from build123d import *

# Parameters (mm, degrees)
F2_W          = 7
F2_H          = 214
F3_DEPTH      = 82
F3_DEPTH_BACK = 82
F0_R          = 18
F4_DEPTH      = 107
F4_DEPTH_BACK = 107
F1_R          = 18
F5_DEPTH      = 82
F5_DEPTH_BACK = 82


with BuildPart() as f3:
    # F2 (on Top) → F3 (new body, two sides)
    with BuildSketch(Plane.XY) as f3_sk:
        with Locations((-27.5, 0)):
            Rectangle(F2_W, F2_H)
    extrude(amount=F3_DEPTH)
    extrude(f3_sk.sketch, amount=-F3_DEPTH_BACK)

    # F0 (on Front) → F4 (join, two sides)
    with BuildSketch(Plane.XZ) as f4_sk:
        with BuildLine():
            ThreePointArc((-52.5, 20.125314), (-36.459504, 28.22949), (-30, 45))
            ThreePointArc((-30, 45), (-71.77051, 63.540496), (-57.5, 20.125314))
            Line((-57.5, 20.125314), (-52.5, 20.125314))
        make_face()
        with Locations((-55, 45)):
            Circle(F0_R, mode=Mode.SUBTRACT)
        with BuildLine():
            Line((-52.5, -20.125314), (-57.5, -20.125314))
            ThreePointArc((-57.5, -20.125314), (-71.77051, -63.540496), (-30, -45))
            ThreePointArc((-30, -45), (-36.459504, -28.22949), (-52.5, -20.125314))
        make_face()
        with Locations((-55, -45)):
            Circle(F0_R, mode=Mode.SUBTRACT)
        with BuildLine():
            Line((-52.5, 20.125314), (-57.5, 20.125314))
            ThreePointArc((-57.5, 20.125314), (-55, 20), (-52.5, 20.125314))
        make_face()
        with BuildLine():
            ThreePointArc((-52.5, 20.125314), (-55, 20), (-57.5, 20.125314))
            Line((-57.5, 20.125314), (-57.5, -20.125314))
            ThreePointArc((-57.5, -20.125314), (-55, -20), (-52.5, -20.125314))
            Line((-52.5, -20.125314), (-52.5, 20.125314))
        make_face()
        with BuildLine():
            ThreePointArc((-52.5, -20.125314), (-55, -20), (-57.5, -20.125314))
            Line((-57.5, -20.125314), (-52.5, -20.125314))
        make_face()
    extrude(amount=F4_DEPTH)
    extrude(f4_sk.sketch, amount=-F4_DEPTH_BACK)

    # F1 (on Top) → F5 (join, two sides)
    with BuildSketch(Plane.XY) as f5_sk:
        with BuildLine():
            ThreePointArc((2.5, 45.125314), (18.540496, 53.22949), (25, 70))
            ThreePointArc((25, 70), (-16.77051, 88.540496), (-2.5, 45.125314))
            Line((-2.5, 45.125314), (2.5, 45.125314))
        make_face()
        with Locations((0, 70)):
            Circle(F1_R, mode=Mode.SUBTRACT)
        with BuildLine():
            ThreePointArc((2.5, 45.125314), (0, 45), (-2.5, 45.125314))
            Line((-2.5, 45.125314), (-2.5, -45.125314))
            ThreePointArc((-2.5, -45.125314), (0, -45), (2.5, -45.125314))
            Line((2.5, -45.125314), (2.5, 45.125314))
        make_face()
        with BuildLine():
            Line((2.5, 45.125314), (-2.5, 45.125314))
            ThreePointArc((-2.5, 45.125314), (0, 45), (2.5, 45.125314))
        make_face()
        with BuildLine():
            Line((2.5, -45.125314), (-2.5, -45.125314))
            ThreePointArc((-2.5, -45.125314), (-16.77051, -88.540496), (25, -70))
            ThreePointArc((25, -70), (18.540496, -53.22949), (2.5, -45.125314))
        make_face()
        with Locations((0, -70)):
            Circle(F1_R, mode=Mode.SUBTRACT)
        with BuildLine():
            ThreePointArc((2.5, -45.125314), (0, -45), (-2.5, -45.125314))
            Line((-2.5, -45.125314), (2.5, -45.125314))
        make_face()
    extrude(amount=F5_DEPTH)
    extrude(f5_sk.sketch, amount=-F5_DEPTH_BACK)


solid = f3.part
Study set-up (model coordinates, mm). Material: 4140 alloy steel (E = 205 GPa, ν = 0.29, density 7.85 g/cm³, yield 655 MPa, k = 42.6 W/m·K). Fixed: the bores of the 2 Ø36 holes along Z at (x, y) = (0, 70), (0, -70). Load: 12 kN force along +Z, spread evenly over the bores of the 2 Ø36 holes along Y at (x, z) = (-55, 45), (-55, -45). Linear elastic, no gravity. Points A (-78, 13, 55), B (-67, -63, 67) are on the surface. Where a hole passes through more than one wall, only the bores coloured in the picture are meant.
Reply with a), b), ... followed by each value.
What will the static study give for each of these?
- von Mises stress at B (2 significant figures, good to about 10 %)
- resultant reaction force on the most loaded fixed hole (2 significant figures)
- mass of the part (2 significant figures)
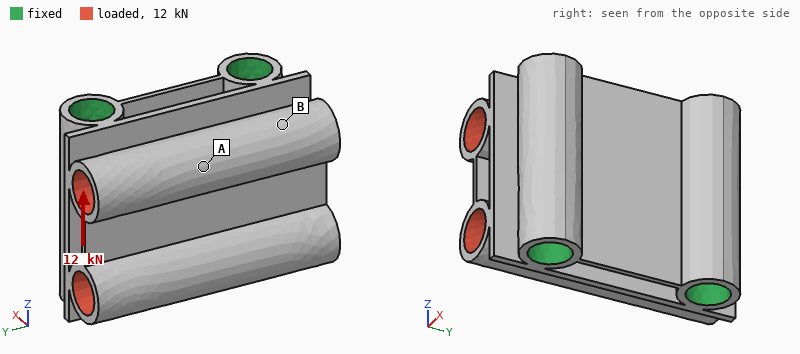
a) 5.0 MPa
b) 6.0 kN
c) 8.4 kg
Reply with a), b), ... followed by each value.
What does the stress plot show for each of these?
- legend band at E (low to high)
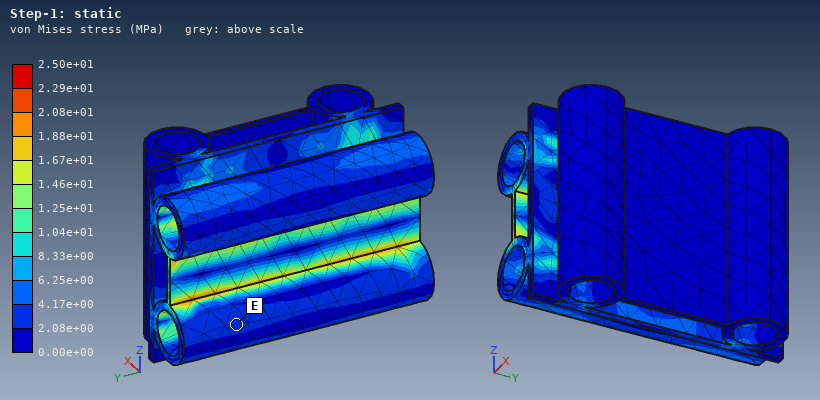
a) 2.08e+00 to 4.17e+00 MPa
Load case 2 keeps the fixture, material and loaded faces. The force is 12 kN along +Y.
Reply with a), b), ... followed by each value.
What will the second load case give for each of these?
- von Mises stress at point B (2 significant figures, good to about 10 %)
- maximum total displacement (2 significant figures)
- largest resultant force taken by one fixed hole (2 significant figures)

a) 1.7 MPa
b) 3.6 µm
c) 6.4 kN
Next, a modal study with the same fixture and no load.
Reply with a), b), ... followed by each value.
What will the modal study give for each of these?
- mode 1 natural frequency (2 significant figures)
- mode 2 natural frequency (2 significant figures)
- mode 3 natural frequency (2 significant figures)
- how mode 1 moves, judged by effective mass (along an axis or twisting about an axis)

a) 2500 Hz
b) 3100 Hz
c) 3300 Hz
d) along Z
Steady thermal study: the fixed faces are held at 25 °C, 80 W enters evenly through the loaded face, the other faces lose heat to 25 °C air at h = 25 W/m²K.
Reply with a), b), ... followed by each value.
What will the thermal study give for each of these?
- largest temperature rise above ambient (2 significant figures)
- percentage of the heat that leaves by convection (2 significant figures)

a) 14 K
b) 37 %
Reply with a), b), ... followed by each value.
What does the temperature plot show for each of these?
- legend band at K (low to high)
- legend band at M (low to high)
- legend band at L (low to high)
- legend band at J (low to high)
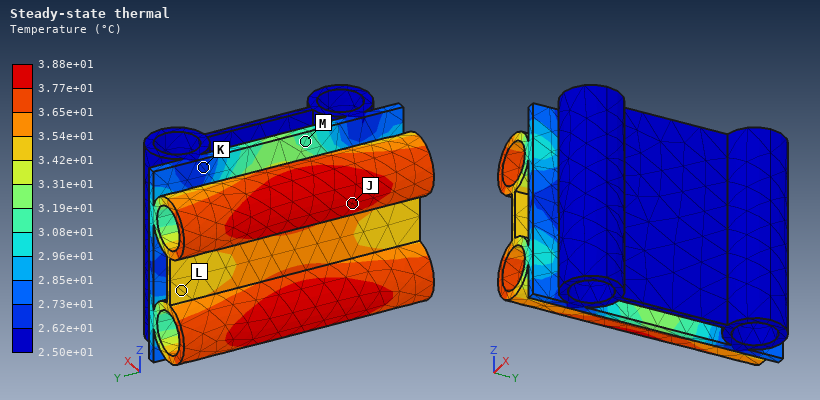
a) 2.62e+01 to 2.73e+01 °C
b) 3.08e+01 to 3.19e+01 °C
c) 3.42e+01 to 3.54e+01 °C
d) 3.77e+01 to 3.88e+01 °C
